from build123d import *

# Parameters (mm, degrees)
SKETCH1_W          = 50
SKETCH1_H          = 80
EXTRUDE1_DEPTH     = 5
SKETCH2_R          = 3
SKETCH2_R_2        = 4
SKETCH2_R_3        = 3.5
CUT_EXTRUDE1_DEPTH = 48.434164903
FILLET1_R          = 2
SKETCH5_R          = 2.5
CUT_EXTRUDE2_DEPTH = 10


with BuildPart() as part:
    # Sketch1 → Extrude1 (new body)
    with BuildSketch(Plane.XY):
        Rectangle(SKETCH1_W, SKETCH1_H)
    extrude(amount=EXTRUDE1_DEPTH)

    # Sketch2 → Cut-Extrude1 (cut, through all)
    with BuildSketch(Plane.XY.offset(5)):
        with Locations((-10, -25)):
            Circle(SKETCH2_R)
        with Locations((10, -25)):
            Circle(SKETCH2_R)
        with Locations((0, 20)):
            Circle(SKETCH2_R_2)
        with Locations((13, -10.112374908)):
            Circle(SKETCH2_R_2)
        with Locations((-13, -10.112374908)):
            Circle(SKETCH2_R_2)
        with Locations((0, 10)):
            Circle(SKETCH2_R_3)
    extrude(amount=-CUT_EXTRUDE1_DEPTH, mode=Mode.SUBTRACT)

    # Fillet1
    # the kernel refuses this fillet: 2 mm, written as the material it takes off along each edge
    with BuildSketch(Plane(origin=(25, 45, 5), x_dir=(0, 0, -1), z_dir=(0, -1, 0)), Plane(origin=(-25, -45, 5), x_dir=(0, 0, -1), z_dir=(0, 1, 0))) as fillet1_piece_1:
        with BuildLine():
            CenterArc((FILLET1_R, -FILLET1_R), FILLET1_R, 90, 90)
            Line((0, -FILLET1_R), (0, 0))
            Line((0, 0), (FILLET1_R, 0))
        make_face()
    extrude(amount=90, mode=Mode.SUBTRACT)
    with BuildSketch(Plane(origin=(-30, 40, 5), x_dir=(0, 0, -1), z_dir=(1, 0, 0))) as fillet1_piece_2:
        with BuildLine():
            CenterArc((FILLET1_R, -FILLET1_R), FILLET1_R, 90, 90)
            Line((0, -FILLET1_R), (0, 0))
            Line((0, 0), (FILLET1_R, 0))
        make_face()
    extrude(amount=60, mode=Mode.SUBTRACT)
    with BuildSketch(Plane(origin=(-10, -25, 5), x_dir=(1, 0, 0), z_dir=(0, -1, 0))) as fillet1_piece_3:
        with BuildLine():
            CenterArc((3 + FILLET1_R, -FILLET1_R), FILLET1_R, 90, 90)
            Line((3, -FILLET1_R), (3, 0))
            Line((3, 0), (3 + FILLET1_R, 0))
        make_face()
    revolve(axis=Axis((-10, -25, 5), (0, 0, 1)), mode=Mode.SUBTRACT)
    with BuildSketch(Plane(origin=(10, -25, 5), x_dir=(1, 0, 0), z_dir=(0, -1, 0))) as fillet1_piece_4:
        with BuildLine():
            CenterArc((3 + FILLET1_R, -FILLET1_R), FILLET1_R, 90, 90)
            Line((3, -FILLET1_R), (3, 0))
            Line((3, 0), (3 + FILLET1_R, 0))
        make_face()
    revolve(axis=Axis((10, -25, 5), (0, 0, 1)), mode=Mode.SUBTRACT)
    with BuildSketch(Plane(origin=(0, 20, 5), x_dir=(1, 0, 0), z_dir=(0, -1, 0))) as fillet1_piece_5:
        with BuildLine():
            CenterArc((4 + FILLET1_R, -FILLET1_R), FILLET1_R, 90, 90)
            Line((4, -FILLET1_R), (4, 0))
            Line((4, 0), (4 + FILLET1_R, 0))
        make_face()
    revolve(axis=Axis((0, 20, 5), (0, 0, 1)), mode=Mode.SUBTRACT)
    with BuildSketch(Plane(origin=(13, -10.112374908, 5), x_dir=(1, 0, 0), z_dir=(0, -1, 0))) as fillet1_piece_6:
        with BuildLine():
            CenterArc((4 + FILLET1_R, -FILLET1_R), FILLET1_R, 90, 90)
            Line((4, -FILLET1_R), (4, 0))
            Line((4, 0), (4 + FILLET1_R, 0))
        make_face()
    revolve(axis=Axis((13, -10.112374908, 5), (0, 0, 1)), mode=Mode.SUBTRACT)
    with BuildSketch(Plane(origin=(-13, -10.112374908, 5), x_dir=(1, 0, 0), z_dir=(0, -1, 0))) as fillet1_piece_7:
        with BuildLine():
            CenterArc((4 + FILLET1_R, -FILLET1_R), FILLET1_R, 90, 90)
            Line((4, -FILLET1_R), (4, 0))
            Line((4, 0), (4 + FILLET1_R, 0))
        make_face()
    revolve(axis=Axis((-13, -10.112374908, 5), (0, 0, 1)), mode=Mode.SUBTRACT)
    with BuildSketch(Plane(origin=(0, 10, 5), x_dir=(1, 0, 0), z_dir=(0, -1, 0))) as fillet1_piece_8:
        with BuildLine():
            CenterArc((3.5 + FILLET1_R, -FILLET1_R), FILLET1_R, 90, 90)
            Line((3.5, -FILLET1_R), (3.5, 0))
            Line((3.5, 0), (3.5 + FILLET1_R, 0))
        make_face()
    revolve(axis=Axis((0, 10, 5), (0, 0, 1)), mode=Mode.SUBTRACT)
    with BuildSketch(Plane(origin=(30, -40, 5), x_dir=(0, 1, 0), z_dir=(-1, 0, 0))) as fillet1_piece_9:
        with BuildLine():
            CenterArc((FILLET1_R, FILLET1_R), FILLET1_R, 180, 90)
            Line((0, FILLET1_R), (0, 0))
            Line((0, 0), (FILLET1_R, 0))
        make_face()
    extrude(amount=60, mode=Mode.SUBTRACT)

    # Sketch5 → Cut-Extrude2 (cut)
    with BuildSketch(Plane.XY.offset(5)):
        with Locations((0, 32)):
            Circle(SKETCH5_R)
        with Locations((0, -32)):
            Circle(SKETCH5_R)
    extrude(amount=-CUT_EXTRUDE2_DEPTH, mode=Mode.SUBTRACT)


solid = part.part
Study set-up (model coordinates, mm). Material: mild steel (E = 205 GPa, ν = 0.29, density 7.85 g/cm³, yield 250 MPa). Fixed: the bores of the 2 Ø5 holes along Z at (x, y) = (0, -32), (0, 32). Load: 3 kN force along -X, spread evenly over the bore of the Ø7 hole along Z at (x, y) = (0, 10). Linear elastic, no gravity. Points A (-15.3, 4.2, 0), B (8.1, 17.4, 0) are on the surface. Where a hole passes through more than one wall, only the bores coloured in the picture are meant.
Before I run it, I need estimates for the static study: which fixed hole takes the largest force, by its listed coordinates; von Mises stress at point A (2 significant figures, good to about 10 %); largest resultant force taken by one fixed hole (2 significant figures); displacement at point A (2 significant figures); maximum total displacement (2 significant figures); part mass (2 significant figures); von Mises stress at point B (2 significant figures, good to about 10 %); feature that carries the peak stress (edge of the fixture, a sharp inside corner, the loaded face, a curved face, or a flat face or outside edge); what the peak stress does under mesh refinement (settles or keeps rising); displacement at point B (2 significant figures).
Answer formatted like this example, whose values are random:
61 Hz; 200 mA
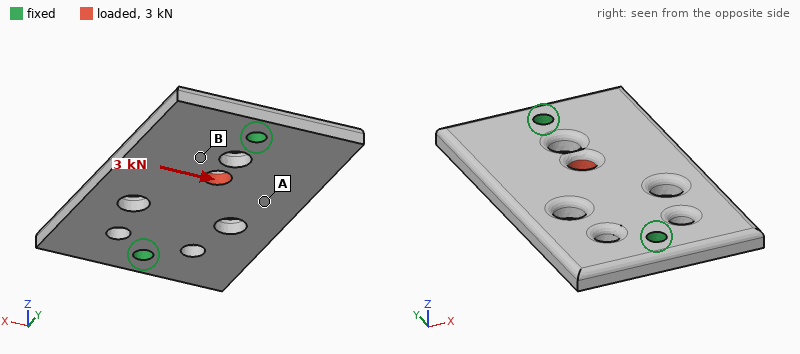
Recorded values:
(0, 32); 10 MPa; 2.0 kN; 6.8 µm; 8.4 µm; 140 g; 30 MPa; edge of the fixture; keeps rising; 4.6 µm
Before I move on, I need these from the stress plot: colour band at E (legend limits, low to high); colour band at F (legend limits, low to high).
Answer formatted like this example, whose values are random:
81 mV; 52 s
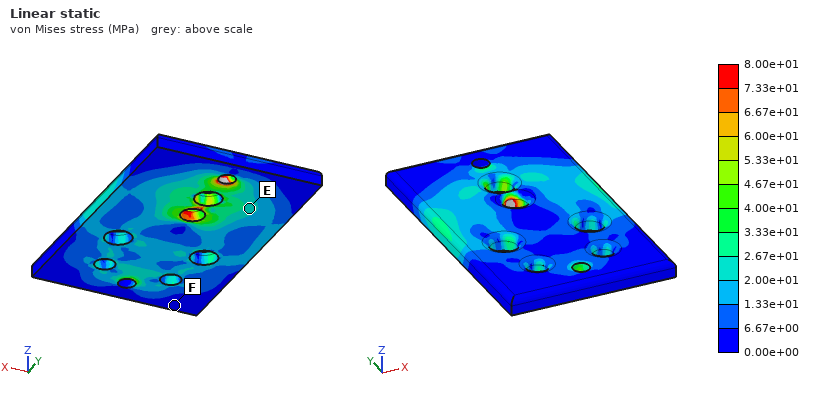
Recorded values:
2.00e+01 to 2.67e+01 MPa; 0.00e+00 to 6.67e+00 MPa
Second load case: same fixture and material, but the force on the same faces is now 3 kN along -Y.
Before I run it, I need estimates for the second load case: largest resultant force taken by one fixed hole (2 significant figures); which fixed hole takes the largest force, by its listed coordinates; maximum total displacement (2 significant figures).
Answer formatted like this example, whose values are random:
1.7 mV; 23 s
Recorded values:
1.6 kN; (0, 32); 5.2 µm
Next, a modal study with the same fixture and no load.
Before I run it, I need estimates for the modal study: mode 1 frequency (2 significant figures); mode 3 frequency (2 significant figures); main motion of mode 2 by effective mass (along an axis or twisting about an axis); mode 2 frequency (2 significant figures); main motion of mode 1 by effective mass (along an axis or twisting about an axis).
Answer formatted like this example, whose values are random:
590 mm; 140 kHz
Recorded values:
3800 Hz; 7200 Hz; along Z; 4300 Hz; twisting about Y
